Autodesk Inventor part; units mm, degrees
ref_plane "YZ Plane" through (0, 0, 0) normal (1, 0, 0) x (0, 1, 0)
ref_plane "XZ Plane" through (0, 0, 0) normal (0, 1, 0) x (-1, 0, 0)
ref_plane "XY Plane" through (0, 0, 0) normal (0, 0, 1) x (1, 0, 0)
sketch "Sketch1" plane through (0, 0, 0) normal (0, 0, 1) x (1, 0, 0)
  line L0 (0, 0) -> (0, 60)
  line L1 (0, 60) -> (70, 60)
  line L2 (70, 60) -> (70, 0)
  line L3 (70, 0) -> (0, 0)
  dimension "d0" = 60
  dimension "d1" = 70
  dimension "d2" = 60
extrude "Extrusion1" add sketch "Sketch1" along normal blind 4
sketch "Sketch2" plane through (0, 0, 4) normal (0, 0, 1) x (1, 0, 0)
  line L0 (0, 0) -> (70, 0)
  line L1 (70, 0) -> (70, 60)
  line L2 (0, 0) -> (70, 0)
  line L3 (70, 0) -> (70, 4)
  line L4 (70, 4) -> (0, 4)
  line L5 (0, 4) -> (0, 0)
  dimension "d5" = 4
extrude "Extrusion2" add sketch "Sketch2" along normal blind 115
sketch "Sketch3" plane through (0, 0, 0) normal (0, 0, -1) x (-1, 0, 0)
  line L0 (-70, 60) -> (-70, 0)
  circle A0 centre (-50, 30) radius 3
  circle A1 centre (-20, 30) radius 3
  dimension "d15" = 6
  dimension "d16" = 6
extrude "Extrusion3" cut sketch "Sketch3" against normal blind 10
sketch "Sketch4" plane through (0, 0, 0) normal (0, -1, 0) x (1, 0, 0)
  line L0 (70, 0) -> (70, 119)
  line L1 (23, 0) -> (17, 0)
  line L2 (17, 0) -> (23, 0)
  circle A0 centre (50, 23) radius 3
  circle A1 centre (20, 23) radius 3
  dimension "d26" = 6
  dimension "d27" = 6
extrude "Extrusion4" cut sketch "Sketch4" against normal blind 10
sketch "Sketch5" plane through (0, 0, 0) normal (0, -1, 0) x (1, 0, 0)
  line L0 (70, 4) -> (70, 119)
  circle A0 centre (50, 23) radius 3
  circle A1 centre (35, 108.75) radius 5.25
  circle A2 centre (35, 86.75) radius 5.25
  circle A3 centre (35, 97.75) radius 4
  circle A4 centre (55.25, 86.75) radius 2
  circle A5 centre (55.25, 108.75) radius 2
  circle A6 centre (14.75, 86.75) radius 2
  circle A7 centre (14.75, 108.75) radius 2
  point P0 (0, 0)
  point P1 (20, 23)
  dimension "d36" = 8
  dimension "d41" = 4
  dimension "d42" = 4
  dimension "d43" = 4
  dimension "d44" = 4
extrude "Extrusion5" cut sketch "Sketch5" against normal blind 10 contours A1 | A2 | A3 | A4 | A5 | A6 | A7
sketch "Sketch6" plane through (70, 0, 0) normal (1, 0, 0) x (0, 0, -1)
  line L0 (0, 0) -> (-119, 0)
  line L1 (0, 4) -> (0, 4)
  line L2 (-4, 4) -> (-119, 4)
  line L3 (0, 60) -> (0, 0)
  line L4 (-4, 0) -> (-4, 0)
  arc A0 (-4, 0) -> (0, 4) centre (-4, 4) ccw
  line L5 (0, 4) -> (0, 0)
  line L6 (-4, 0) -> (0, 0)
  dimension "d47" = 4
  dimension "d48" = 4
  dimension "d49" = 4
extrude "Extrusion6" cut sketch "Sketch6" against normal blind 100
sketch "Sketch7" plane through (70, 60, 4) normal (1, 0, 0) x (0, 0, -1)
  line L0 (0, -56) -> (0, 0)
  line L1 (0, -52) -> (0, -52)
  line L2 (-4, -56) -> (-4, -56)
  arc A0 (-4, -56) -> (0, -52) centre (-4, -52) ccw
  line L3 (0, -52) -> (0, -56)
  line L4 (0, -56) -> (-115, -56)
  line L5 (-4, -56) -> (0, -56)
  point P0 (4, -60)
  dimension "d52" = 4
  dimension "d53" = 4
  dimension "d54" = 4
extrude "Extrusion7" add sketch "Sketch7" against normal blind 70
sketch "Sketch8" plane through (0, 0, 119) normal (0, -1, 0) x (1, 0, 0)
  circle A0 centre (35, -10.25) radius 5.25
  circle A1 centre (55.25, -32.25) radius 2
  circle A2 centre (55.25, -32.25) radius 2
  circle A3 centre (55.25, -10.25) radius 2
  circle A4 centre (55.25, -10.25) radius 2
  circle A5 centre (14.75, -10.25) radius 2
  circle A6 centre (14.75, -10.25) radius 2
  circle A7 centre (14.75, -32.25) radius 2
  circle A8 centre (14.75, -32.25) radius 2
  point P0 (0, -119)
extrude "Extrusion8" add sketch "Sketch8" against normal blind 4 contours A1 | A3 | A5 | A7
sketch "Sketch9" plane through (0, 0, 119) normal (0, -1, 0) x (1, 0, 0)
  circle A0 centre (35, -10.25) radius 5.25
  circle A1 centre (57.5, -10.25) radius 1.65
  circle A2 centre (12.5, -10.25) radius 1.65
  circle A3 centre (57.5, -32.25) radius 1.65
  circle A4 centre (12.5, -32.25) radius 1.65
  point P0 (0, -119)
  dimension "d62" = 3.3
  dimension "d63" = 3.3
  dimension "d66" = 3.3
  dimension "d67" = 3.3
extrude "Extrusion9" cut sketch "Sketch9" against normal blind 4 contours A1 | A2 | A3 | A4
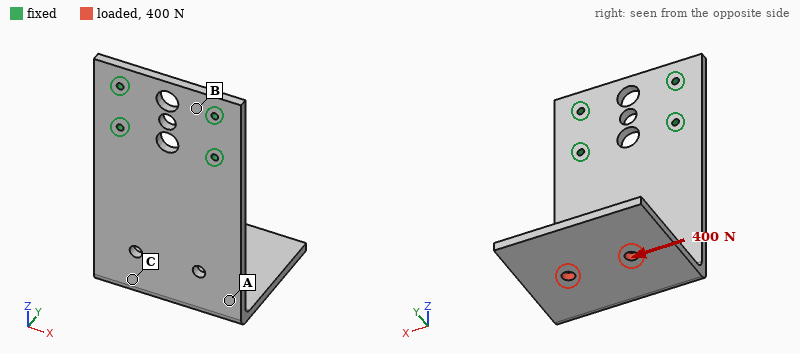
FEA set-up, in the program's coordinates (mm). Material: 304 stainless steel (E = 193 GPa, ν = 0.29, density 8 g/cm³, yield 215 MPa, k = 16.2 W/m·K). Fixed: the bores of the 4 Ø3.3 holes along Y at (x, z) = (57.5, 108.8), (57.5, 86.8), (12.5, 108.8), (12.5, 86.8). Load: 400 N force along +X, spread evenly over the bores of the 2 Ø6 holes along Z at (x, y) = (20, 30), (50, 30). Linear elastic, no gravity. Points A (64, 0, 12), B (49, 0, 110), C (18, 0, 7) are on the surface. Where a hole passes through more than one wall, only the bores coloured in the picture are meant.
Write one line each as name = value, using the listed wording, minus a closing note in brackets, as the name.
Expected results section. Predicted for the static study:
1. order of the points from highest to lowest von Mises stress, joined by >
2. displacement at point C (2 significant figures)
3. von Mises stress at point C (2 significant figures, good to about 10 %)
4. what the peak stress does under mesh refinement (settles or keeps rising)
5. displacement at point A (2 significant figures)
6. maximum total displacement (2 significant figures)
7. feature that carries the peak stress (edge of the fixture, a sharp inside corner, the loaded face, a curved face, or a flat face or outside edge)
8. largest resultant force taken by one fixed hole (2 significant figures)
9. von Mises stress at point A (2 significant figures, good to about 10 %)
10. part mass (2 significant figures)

order of the points from highest to lowest von Mises stress, joined by > = A > C > B
displacement at point C = 0.099 mm
von Mises stress at point C = 31 MPa
what the peak stress does under mesh refinement = keeps rising
displacement at point A = 0.17 mm
maximum total displacement = 0.43 mm
feature that carries the peak stress = edge of the fixture
largest resultant force taken by one fixed hole = 650 N
von Mises stress at point A = 41 MPa
part mass = 380 g
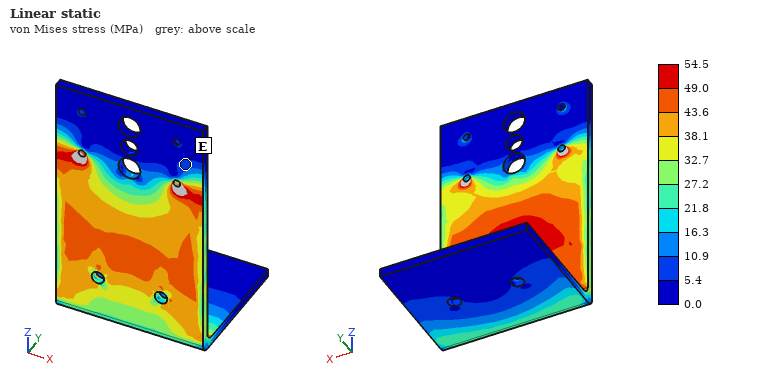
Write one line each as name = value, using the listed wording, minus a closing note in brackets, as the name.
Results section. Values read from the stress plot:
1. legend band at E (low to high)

legend band at E = 5.4 to 10.9 MPa
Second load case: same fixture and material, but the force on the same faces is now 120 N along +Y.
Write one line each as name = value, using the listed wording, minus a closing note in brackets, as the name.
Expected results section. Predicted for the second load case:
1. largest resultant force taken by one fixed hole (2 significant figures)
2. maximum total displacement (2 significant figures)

largest resultant force taken by one fixed hole = 160 N
maximum total displacement = 0.53 mm
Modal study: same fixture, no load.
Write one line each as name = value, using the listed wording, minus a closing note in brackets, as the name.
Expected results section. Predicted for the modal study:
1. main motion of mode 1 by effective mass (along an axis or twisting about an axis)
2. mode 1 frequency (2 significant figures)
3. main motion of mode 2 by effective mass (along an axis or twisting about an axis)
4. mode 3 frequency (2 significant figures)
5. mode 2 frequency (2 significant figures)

main motion of mode 1 by effective mass = along Y
mode 1 frequency = 190 Hz
main motion of mode 2 by effective mass = along X
mode 3 frequency = 680 Hz
mode 2 frequency = 450 Hz
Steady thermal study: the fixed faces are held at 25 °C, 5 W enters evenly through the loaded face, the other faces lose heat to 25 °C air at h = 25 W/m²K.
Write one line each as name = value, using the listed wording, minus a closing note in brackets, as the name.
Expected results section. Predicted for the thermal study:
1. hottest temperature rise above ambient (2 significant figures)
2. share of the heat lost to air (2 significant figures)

hottest temperature rise above ambient = 27 K
share of the heat lost to air = 96 %
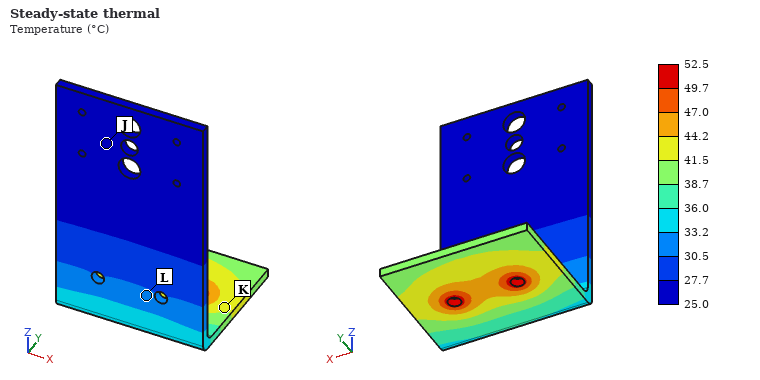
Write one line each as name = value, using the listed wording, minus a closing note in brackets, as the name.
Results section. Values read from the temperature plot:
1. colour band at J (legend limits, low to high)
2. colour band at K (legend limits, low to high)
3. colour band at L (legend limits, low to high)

colour band at J = 25.0 to 27.7 °C
colour band at K = 41.5 to 44.2 °C
colour band at L = 30.5 to 33.2 °C
